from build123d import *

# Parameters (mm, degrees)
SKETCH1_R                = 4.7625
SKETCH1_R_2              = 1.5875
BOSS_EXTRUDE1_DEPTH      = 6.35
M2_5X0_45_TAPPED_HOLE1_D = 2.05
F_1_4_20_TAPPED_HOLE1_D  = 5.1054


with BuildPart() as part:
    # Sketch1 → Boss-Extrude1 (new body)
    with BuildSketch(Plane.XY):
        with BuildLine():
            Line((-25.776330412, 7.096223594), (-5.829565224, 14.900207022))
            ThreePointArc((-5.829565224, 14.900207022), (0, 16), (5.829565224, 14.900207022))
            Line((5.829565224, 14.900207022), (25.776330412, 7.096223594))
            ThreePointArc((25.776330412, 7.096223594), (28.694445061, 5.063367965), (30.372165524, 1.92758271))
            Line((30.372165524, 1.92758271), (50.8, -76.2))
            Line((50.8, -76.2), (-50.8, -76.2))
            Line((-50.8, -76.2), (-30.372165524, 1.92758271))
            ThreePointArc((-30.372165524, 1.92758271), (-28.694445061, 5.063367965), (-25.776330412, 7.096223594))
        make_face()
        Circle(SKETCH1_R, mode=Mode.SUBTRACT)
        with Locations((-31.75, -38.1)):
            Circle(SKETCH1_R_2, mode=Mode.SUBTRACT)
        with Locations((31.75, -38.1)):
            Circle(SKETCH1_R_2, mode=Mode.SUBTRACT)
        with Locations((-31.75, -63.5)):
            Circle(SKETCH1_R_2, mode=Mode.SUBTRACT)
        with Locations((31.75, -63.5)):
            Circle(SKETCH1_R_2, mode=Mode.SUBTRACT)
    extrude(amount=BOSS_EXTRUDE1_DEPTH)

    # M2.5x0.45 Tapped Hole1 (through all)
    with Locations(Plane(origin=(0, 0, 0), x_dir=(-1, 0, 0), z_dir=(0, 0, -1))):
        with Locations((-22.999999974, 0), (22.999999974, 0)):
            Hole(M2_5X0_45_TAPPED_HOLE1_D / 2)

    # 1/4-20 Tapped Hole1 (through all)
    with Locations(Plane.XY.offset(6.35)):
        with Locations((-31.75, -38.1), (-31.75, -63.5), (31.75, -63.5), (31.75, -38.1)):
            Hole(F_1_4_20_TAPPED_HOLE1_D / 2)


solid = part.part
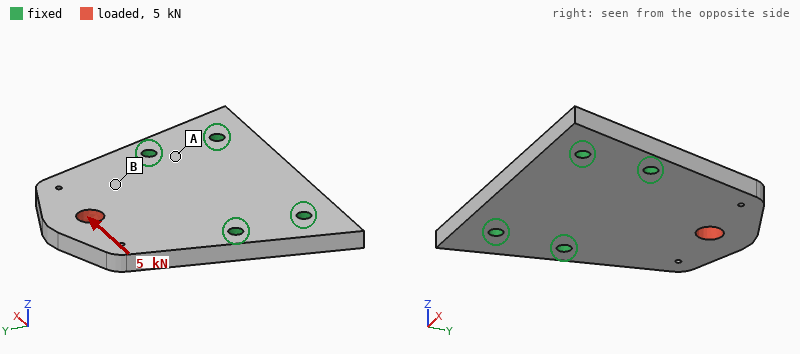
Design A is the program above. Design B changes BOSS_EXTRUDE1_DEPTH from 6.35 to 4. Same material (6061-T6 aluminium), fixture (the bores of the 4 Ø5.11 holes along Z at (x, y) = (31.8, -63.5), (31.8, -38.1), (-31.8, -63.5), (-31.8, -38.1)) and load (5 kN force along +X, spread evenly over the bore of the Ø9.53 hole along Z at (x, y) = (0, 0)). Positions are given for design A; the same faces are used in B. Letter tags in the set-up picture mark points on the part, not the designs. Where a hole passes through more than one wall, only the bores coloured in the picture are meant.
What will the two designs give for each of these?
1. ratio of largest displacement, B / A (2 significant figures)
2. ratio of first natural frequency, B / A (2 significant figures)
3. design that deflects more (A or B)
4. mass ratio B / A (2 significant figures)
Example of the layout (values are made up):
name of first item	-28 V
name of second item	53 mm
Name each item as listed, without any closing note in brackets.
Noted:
ratio of largest displacement, B / A	1.6
ratio of first natural frequency, B / A	0.65
design that deflects more	B
mass ratio B / A	0.63
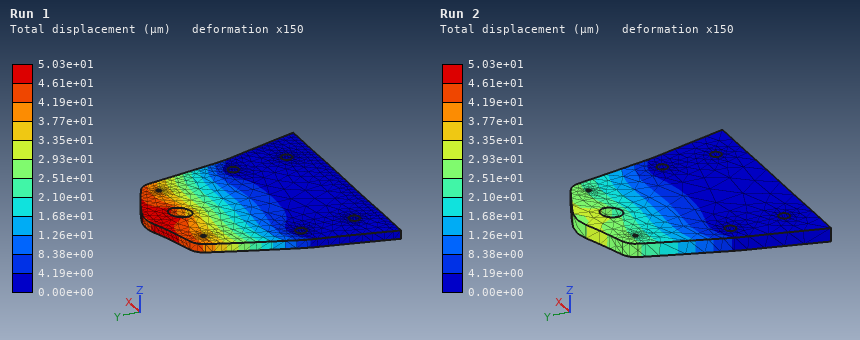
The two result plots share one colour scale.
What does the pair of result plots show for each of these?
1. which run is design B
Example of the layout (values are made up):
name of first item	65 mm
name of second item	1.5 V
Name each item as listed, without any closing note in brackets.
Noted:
which run is design B	Run 1
